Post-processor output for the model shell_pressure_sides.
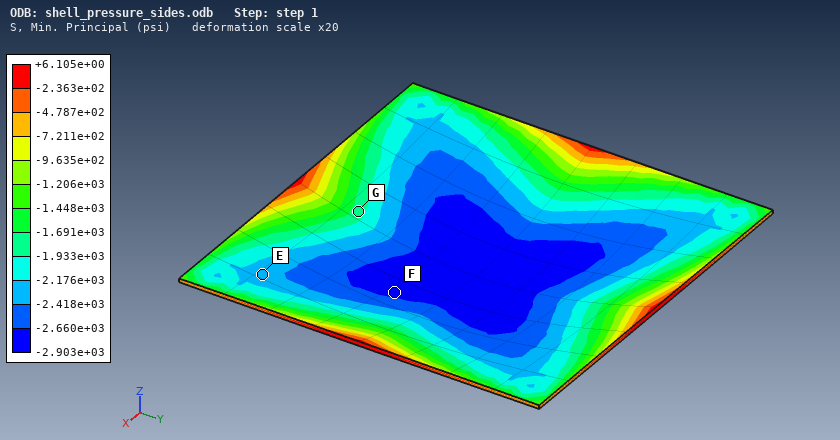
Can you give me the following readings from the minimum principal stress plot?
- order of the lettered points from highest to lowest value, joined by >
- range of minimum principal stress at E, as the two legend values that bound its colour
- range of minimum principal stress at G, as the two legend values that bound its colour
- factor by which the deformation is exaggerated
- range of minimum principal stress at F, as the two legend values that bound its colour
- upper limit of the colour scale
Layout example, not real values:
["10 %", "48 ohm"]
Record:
["G > E > F", "-2.418e+03 to -2.176e+03 psi", "-1.933e+03 to -1.691e+03 psi", "20", "-2.903e+03 to -2.660e+03 psi", "+6.105e+00 psi"]
